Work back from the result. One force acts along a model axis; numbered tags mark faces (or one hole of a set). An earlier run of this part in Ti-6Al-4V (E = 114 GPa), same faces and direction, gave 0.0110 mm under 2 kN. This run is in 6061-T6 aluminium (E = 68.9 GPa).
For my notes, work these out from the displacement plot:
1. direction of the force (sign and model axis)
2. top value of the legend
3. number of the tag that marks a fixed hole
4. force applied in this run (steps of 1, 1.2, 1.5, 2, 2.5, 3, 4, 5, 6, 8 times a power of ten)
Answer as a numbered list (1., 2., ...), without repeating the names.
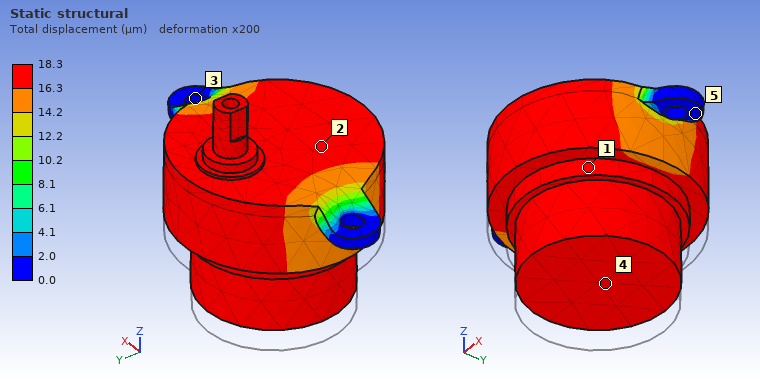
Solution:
1. +Z
2. 18.3 µm
3. 3
4. 2 kN
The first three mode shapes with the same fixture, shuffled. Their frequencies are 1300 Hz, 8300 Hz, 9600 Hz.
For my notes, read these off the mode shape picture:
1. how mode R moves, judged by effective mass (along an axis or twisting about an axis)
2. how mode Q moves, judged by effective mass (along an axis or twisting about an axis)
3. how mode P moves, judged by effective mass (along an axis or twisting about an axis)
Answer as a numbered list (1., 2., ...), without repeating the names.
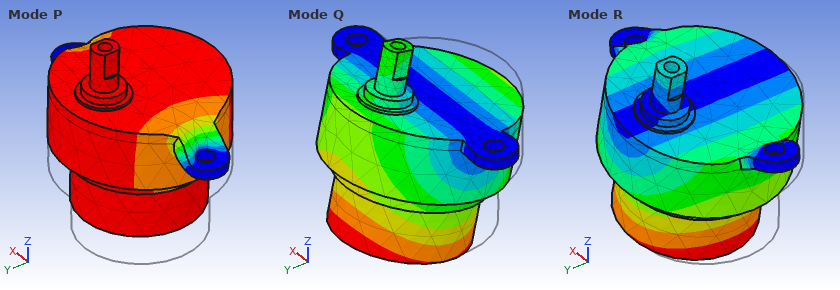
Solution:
1. along X
2. along Y
3. along Z
